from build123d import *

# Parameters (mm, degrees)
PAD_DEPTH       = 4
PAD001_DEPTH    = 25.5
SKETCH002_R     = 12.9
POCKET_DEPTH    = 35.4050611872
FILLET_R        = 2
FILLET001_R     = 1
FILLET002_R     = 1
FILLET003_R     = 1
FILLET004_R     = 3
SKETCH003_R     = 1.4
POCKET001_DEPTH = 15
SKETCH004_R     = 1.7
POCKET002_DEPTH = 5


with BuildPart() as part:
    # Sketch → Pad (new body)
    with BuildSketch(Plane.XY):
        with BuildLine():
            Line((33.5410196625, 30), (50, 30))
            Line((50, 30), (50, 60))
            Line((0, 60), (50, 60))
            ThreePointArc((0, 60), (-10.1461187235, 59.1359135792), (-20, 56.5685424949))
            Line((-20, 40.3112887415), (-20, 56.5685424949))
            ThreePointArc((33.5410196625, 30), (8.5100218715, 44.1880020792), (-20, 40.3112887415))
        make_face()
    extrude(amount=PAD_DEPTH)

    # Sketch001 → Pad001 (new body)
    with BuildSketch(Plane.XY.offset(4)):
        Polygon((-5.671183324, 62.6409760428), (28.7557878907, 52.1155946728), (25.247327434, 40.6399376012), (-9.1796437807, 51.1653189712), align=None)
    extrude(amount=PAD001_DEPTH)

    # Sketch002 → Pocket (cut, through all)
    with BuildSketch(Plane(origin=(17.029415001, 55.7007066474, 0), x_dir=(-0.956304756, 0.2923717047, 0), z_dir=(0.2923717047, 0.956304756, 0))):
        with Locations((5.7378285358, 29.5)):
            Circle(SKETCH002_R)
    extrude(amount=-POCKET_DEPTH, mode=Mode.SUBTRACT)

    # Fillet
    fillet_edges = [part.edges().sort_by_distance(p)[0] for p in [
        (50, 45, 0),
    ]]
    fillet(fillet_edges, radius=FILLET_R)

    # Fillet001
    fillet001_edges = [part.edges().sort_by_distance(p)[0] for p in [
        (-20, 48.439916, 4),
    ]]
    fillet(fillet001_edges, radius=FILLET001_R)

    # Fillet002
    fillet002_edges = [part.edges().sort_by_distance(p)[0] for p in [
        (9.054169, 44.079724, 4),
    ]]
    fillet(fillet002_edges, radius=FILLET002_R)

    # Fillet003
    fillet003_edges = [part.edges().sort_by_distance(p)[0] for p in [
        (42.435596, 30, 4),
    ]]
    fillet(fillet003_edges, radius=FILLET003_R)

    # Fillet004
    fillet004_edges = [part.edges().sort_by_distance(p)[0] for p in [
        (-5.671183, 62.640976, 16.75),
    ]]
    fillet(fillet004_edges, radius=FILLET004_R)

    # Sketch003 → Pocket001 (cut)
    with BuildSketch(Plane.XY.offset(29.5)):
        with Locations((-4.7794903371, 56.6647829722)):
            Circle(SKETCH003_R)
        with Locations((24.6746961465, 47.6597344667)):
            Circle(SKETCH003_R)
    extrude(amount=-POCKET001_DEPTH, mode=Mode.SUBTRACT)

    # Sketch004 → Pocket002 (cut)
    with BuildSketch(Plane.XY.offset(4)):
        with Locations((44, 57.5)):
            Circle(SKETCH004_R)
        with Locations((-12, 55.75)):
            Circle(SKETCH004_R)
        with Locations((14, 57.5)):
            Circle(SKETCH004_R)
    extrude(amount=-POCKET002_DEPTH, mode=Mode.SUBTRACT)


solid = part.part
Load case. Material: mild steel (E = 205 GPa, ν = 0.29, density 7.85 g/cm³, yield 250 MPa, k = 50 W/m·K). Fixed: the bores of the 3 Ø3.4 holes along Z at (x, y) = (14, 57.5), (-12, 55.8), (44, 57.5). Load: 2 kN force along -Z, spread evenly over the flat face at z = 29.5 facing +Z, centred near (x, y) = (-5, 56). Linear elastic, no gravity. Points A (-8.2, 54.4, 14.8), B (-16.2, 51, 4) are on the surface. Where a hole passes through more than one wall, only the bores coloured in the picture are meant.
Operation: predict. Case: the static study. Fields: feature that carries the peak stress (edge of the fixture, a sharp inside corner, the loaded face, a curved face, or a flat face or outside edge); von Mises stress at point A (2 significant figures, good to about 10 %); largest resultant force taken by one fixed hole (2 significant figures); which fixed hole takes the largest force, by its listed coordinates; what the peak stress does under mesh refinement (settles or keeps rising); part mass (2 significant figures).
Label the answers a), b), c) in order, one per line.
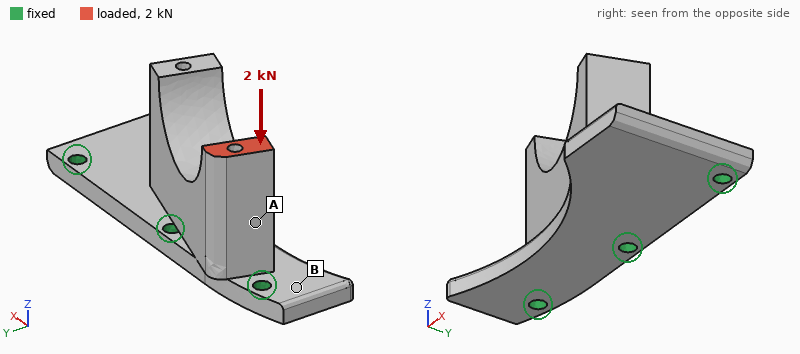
a) edge of the fixture
b) 42 MPa
c) 1.5 kN
d) (-12, 55.8)
e) keeps rising
f) 100 g
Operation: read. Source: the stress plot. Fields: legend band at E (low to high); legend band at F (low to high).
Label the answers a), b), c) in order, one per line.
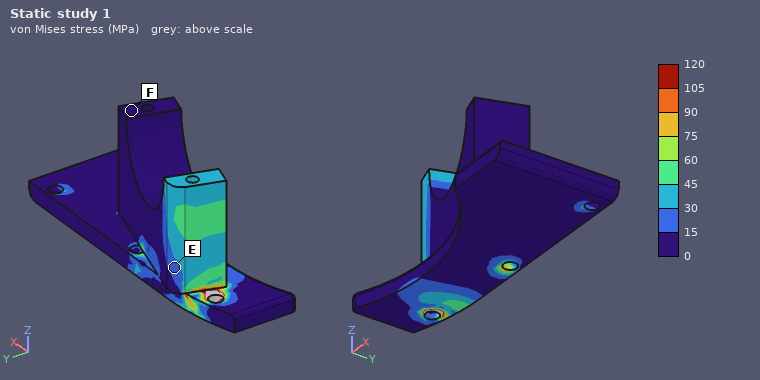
a) 15 to 30 MPa
b) 0 to 15 MPa
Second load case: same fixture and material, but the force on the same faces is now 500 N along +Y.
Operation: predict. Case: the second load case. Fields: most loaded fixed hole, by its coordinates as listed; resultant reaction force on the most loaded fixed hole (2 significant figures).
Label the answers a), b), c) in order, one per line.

a) (14, 57.5)
b) 490 N
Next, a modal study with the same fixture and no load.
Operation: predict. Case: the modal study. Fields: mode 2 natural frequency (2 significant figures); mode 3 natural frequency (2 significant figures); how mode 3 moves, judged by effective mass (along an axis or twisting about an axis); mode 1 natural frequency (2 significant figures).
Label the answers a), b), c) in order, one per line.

a) 7300 Hz
b) 12 kHz
c) along X
d) 3900 Hz
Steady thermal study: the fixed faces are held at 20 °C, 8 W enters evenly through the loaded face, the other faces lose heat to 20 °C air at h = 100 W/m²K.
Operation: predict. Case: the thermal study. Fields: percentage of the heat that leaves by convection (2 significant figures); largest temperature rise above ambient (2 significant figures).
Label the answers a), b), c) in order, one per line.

a) 38 %
b) 41 K
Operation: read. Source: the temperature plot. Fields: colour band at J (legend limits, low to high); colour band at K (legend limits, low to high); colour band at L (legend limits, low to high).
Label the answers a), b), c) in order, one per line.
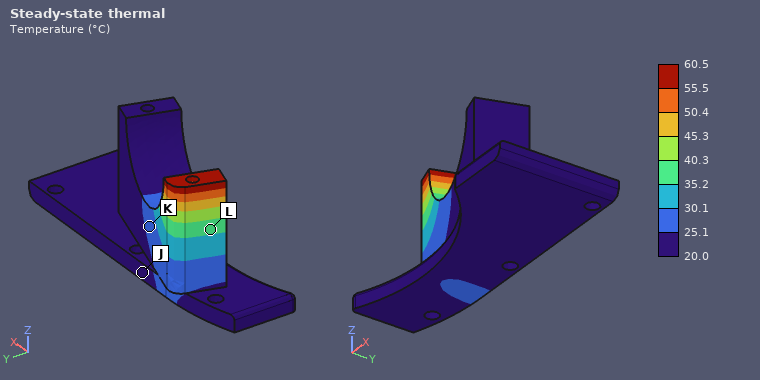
a) 20.0 to 25.1 °C
b) 25.1 to 30.1 °C
c) 35.2 to 40.3 °C
